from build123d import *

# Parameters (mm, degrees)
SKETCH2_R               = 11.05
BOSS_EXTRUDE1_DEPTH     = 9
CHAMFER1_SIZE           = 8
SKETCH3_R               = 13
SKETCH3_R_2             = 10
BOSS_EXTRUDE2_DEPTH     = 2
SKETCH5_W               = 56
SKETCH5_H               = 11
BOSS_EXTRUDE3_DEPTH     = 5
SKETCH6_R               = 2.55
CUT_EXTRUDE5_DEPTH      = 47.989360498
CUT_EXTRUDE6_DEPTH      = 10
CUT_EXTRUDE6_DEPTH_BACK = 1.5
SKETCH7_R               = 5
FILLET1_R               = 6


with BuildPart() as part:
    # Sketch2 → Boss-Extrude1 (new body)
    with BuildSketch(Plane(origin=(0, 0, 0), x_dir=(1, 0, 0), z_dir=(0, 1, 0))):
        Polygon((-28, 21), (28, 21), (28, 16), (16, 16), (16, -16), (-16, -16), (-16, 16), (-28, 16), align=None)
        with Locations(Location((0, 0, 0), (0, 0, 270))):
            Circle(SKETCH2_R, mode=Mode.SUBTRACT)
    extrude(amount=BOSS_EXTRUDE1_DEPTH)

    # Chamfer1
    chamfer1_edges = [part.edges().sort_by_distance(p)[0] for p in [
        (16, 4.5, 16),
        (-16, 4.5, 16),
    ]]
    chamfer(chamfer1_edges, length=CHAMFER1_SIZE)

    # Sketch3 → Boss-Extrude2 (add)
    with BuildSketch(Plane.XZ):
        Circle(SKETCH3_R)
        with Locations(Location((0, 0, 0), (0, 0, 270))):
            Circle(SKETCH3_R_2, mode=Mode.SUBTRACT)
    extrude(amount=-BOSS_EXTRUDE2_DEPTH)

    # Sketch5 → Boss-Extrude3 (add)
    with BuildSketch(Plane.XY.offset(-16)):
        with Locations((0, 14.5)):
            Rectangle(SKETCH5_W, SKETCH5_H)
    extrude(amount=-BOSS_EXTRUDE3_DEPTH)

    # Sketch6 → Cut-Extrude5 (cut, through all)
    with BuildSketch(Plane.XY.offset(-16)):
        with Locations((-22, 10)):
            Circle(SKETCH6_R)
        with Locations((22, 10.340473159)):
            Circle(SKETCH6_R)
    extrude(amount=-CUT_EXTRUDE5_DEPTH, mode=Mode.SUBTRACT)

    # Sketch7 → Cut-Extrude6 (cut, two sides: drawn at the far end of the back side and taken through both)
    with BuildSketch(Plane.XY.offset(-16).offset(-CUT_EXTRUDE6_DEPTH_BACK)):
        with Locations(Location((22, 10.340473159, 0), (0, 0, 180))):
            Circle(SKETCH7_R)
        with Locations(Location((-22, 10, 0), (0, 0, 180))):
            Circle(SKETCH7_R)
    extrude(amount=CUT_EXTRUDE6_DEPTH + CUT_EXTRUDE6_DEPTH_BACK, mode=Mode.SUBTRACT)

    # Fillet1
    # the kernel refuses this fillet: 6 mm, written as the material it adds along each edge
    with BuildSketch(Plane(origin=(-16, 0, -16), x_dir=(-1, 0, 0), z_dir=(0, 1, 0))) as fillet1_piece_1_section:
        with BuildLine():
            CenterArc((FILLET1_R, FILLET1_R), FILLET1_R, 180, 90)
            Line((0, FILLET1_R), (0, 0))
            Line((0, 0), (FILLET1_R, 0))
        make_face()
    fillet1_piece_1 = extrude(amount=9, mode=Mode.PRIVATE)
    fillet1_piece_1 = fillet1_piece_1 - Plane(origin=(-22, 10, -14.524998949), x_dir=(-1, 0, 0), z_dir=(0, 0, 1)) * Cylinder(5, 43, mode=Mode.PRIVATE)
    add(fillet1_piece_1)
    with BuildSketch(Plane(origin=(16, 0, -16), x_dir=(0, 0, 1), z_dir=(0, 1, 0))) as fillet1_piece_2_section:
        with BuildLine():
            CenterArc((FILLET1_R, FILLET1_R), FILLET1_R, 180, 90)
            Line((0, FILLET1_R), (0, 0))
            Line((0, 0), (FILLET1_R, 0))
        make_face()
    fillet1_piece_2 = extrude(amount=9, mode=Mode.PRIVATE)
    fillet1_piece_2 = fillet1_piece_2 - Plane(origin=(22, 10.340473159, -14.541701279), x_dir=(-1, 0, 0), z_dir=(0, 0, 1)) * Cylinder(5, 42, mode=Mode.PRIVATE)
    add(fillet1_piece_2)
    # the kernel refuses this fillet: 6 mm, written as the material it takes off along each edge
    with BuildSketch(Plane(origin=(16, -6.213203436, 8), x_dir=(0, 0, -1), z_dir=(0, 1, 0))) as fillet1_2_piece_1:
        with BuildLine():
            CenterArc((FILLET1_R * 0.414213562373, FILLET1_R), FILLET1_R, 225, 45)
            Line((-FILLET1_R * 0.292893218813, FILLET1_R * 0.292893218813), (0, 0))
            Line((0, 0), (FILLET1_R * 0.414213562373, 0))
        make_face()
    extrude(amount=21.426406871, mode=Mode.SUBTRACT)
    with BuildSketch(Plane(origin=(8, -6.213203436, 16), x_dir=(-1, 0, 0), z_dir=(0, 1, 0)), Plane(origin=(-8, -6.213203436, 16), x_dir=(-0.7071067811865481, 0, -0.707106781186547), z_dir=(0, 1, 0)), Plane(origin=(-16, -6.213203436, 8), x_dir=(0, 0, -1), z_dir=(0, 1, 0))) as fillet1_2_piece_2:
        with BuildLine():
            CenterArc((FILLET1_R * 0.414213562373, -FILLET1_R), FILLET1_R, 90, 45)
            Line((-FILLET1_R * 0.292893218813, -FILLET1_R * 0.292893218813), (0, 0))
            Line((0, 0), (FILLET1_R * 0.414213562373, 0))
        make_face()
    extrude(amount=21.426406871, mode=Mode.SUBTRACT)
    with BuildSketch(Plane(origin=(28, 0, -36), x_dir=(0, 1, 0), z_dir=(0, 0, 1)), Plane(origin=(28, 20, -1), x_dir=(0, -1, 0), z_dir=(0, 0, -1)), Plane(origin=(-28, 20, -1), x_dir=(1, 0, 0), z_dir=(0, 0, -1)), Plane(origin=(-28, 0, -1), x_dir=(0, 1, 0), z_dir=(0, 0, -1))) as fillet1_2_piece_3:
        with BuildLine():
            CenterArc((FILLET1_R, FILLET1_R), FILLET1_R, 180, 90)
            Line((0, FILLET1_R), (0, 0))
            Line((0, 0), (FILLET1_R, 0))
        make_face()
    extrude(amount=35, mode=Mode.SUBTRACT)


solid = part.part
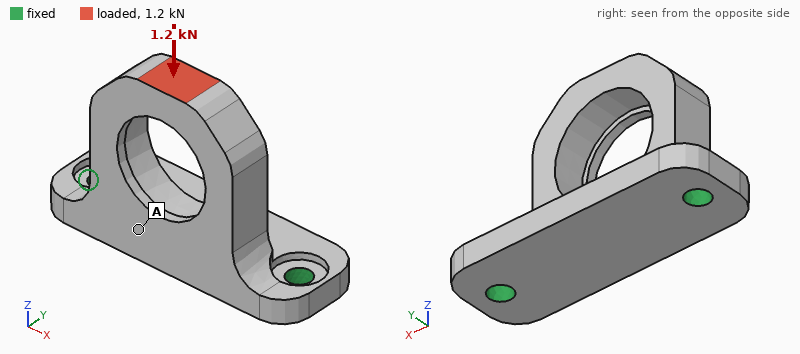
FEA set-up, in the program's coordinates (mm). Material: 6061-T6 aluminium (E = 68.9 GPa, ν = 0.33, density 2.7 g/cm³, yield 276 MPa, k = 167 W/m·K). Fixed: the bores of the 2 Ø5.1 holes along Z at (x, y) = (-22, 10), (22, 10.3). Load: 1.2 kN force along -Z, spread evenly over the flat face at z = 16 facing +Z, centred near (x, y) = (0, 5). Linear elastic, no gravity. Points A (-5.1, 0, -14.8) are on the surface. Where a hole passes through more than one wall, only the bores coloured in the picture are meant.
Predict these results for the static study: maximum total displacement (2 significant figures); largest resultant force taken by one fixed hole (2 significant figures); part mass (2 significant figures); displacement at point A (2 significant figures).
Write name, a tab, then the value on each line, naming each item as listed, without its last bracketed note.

maximum total displacement	58 µm
largest resultant force taken by one fixed hole	650 N
part mass	28 g
displacement at point A	18 µm
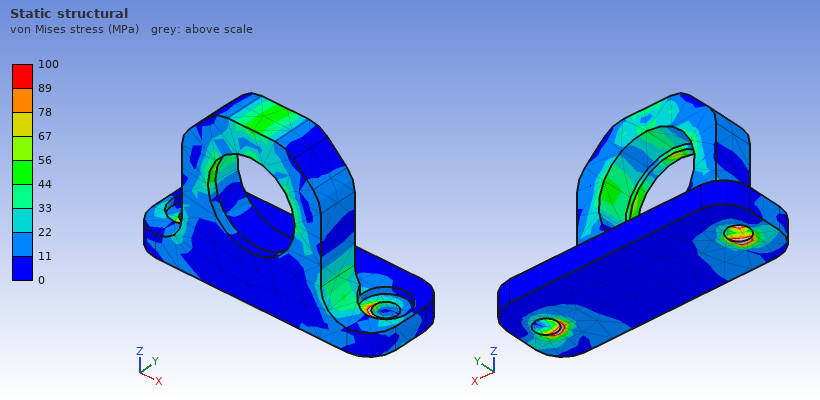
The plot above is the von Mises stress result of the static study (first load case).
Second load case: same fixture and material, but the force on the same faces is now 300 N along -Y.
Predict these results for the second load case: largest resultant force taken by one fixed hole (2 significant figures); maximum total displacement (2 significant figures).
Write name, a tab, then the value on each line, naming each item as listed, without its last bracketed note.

largest resultant force taken by one fixed hole	160 N
maximum total displacement	0.18 mm
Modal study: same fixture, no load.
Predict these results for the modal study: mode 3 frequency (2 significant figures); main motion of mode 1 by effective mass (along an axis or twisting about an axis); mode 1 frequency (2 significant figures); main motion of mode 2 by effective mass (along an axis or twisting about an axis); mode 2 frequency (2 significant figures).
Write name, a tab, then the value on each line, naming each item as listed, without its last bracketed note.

mode 3 frequency	11 kHz
main motion of mode 1 by effective mass	along Y
mode 1 frequency	3100 Hz
main motion of mode 2 by effective mass	along X
mode 2 frequency	8400 Hz
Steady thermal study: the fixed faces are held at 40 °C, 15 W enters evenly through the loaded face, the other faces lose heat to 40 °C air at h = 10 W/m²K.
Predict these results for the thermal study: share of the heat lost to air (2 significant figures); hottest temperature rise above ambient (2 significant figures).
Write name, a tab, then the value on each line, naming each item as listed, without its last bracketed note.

share of the heat lost to air	3.3 %
hottest temperature rise above ambient	33 K
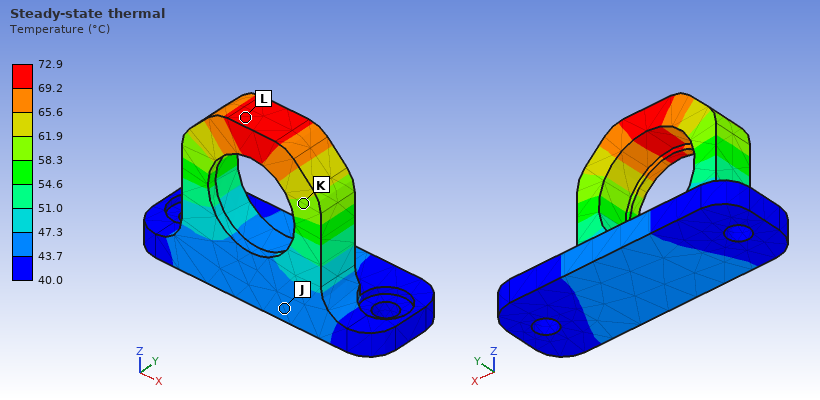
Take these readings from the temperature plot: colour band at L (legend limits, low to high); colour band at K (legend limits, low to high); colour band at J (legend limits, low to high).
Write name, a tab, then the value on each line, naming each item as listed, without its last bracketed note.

colour band at L	69.2 to 72.9 °C
colour band at K	58.3 to 61.9 °C
colour band at J	43.7 to 47.3 °C
